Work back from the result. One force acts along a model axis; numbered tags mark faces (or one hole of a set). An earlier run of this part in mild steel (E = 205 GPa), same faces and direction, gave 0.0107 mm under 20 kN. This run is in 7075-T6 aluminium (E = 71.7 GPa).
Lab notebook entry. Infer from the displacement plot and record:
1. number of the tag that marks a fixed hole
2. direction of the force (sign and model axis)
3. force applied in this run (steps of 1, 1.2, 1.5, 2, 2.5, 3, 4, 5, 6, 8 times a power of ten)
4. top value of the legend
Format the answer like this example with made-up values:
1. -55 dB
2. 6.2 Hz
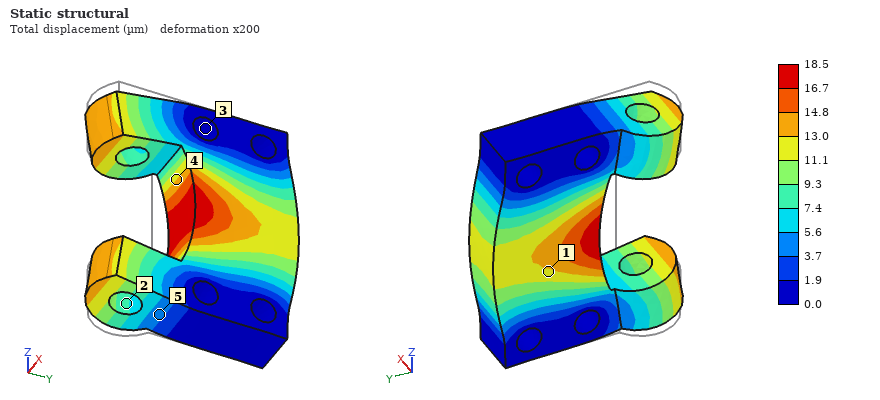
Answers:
1. 3
2. +Y
3. 12 kN
4. 18.5 µm
